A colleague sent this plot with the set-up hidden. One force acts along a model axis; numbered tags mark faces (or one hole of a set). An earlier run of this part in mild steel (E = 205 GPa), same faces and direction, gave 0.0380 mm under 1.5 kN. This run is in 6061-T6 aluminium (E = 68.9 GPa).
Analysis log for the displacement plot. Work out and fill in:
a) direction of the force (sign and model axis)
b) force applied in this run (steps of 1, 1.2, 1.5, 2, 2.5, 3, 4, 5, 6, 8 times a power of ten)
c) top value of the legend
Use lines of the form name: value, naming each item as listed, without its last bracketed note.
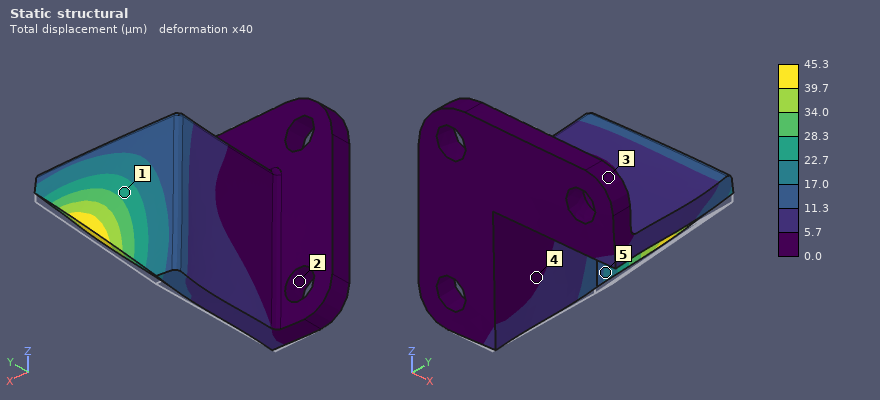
direction of the force: +Y
force applied in this run: 600 N
top value of the legend: 45.3 µm
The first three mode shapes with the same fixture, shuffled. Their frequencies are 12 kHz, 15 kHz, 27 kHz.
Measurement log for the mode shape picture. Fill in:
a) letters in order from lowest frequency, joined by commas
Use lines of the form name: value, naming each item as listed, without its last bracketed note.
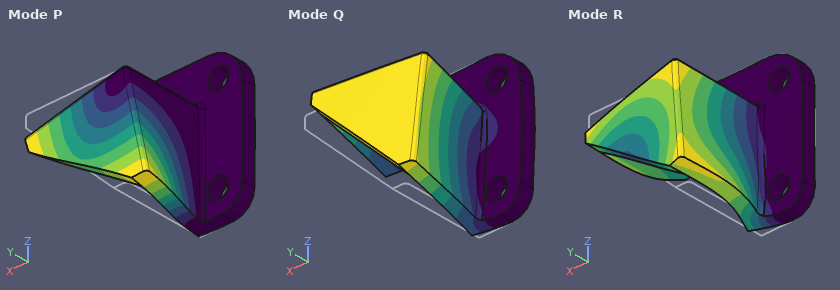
letters in order from lowest frequency, joined by commas: P, Q, R
